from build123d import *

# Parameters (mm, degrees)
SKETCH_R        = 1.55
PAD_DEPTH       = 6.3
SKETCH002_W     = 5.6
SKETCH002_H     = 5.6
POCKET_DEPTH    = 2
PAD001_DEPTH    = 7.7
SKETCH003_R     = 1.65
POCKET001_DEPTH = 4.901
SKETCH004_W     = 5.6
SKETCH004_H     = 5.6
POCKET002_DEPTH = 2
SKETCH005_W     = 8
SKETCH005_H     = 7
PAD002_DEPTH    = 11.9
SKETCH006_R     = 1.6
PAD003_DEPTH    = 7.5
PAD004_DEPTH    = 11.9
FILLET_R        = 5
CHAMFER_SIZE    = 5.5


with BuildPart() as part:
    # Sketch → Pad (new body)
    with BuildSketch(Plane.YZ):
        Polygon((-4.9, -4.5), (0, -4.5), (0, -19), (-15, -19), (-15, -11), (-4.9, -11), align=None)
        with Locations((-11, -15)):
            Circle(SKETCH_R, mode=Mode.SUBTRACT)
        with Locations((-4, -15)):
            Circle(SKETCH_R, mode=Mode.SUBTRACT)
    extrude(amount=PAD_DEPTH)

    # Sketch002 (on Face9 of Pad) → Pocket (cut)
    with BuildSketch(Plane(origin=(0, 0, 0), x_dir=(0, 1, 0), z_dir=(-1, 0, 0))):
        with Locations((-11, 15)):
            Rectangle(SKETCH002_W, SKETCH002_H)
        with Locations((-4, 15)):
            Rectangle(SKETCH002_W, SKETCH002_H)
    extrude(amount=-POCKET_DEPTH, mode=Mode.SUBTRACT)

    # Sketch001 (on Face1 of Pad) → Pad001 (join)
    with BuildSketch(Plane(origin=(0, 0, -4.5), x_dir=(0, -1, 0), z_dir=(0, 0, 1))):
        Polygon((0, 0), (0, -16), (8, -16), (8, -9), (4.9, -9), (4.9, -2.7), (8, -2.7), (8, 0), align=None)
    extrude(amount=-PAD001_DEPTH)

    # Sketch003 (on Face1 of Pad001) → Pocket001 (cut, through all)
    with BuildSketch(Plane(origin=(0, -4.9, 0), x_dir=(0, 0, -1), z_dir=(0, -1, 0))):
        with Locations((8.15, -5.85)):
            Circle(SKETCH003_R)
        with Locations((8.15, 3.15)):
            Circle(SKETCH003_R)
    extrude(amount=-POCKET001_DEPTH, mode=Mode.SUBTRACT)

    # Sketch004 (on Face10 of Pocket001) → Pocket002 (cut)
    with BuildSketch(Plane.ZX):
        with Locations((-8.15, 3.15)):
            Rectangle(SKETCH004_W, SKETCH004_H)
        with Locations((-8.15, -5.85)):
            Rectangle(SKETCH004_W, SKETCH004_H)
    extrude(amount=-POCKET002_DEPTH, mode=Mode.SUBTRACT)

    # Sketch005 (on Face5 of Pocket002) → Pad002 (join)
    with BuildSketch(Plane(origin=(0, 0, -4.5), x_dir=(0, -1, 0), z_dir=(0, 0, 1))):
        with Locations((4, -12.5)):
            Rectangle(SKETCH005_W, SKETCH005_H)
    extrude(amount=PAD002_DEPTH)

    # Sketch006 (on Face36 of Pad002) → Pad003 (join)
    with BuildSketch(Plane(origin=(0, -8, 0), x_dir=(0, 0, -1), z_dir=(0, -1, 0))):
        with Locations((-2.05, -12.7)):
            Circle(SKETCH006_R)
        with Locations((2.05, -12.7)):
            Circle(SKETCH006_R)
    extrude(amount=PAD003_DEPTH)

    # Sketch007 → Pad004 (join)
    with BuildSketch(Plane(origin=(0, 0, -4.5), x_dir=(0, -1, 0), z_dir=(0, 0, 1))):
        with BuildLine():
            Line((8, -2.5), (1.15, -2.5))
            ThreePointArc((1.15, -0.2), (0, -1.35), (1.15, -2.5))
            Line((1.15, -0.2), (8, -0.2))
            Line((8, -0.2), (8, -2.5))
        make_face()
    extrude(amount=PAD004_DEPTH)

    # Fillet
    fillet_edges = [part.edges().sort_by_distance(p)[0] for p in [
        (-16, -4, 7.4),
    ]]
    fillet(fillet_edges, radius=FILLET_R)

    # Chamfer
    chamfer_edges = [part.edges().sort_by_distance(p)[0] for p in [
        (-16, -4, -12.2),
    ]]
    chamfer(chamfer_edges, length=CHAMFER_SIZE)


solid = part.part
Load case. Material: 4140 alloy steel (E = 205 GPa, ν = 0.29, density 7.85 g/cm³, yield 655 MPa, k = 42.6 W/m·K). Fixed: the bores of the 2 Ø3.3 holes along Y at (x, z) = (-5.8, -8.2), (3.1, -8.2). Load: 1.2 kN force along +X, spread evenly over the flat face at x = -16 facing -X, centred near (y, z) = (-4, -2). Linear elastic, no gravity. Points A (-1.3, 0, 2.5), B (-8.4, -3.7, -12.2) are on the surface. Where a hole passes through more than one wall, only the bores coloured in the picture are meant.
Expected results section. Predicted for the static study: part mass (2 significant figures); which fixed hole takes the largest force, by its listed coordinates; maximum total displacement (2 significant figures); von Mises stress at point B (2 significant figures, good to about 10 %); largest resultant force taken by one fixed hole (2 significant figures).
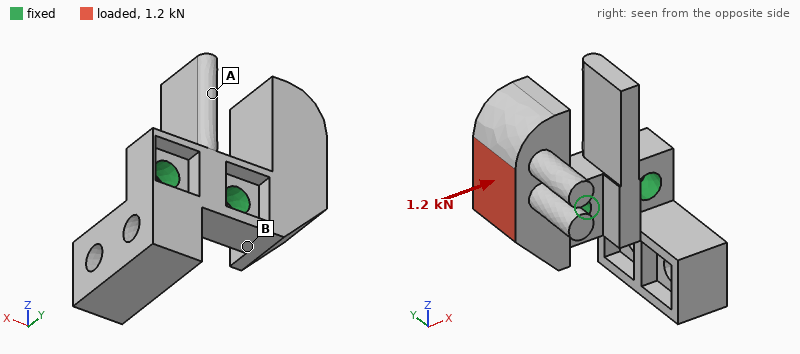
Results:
18 g
(-5.8, -8.2)
36 µm
97 MPa
1.2 kN
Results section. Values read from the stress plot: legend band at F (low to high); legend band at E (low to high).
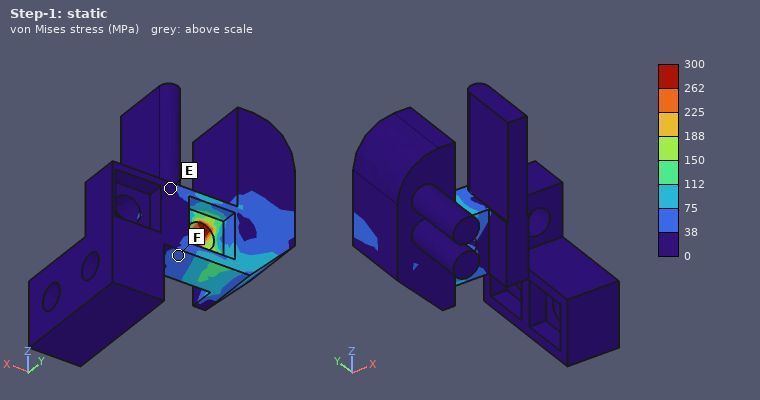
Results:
38 to 75 MPa
0 to 38 MPa
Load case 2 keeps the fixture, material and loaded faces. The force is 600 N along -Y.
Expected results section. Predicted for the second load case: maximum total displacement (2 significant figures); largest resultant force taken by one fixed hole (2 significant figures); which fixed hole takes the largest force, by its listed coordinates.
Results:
60 µm
810 N
(-5.8, -8.2)
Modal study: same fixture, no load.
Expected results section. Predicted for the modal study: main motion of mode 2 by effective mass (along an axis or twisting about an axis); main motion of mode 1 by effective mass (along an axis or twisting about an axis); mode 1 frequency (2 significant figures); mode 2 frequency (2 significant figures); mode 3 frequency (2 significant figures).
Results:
along X
along Y
7700 Hz
10 kHz
11 kHz
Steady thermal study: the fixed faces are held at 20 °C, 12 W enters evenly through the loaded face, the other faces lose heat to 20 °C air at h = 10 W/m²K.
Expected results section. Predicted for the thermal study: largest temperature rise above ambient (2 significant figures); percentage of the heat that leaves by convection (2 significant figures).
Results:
73 K
3.4 %
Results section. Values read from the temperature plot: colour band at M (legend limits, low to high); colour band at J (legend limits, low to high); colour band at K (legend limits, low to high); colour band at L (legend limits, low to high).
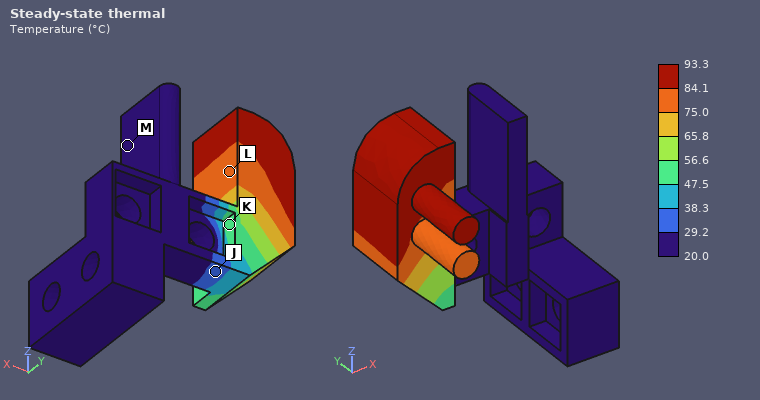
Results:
20.0 to 29.2 °C
29.2 to 38.3 °C
47.5 to 56.6 °C
75.0 to 84.1 °C
